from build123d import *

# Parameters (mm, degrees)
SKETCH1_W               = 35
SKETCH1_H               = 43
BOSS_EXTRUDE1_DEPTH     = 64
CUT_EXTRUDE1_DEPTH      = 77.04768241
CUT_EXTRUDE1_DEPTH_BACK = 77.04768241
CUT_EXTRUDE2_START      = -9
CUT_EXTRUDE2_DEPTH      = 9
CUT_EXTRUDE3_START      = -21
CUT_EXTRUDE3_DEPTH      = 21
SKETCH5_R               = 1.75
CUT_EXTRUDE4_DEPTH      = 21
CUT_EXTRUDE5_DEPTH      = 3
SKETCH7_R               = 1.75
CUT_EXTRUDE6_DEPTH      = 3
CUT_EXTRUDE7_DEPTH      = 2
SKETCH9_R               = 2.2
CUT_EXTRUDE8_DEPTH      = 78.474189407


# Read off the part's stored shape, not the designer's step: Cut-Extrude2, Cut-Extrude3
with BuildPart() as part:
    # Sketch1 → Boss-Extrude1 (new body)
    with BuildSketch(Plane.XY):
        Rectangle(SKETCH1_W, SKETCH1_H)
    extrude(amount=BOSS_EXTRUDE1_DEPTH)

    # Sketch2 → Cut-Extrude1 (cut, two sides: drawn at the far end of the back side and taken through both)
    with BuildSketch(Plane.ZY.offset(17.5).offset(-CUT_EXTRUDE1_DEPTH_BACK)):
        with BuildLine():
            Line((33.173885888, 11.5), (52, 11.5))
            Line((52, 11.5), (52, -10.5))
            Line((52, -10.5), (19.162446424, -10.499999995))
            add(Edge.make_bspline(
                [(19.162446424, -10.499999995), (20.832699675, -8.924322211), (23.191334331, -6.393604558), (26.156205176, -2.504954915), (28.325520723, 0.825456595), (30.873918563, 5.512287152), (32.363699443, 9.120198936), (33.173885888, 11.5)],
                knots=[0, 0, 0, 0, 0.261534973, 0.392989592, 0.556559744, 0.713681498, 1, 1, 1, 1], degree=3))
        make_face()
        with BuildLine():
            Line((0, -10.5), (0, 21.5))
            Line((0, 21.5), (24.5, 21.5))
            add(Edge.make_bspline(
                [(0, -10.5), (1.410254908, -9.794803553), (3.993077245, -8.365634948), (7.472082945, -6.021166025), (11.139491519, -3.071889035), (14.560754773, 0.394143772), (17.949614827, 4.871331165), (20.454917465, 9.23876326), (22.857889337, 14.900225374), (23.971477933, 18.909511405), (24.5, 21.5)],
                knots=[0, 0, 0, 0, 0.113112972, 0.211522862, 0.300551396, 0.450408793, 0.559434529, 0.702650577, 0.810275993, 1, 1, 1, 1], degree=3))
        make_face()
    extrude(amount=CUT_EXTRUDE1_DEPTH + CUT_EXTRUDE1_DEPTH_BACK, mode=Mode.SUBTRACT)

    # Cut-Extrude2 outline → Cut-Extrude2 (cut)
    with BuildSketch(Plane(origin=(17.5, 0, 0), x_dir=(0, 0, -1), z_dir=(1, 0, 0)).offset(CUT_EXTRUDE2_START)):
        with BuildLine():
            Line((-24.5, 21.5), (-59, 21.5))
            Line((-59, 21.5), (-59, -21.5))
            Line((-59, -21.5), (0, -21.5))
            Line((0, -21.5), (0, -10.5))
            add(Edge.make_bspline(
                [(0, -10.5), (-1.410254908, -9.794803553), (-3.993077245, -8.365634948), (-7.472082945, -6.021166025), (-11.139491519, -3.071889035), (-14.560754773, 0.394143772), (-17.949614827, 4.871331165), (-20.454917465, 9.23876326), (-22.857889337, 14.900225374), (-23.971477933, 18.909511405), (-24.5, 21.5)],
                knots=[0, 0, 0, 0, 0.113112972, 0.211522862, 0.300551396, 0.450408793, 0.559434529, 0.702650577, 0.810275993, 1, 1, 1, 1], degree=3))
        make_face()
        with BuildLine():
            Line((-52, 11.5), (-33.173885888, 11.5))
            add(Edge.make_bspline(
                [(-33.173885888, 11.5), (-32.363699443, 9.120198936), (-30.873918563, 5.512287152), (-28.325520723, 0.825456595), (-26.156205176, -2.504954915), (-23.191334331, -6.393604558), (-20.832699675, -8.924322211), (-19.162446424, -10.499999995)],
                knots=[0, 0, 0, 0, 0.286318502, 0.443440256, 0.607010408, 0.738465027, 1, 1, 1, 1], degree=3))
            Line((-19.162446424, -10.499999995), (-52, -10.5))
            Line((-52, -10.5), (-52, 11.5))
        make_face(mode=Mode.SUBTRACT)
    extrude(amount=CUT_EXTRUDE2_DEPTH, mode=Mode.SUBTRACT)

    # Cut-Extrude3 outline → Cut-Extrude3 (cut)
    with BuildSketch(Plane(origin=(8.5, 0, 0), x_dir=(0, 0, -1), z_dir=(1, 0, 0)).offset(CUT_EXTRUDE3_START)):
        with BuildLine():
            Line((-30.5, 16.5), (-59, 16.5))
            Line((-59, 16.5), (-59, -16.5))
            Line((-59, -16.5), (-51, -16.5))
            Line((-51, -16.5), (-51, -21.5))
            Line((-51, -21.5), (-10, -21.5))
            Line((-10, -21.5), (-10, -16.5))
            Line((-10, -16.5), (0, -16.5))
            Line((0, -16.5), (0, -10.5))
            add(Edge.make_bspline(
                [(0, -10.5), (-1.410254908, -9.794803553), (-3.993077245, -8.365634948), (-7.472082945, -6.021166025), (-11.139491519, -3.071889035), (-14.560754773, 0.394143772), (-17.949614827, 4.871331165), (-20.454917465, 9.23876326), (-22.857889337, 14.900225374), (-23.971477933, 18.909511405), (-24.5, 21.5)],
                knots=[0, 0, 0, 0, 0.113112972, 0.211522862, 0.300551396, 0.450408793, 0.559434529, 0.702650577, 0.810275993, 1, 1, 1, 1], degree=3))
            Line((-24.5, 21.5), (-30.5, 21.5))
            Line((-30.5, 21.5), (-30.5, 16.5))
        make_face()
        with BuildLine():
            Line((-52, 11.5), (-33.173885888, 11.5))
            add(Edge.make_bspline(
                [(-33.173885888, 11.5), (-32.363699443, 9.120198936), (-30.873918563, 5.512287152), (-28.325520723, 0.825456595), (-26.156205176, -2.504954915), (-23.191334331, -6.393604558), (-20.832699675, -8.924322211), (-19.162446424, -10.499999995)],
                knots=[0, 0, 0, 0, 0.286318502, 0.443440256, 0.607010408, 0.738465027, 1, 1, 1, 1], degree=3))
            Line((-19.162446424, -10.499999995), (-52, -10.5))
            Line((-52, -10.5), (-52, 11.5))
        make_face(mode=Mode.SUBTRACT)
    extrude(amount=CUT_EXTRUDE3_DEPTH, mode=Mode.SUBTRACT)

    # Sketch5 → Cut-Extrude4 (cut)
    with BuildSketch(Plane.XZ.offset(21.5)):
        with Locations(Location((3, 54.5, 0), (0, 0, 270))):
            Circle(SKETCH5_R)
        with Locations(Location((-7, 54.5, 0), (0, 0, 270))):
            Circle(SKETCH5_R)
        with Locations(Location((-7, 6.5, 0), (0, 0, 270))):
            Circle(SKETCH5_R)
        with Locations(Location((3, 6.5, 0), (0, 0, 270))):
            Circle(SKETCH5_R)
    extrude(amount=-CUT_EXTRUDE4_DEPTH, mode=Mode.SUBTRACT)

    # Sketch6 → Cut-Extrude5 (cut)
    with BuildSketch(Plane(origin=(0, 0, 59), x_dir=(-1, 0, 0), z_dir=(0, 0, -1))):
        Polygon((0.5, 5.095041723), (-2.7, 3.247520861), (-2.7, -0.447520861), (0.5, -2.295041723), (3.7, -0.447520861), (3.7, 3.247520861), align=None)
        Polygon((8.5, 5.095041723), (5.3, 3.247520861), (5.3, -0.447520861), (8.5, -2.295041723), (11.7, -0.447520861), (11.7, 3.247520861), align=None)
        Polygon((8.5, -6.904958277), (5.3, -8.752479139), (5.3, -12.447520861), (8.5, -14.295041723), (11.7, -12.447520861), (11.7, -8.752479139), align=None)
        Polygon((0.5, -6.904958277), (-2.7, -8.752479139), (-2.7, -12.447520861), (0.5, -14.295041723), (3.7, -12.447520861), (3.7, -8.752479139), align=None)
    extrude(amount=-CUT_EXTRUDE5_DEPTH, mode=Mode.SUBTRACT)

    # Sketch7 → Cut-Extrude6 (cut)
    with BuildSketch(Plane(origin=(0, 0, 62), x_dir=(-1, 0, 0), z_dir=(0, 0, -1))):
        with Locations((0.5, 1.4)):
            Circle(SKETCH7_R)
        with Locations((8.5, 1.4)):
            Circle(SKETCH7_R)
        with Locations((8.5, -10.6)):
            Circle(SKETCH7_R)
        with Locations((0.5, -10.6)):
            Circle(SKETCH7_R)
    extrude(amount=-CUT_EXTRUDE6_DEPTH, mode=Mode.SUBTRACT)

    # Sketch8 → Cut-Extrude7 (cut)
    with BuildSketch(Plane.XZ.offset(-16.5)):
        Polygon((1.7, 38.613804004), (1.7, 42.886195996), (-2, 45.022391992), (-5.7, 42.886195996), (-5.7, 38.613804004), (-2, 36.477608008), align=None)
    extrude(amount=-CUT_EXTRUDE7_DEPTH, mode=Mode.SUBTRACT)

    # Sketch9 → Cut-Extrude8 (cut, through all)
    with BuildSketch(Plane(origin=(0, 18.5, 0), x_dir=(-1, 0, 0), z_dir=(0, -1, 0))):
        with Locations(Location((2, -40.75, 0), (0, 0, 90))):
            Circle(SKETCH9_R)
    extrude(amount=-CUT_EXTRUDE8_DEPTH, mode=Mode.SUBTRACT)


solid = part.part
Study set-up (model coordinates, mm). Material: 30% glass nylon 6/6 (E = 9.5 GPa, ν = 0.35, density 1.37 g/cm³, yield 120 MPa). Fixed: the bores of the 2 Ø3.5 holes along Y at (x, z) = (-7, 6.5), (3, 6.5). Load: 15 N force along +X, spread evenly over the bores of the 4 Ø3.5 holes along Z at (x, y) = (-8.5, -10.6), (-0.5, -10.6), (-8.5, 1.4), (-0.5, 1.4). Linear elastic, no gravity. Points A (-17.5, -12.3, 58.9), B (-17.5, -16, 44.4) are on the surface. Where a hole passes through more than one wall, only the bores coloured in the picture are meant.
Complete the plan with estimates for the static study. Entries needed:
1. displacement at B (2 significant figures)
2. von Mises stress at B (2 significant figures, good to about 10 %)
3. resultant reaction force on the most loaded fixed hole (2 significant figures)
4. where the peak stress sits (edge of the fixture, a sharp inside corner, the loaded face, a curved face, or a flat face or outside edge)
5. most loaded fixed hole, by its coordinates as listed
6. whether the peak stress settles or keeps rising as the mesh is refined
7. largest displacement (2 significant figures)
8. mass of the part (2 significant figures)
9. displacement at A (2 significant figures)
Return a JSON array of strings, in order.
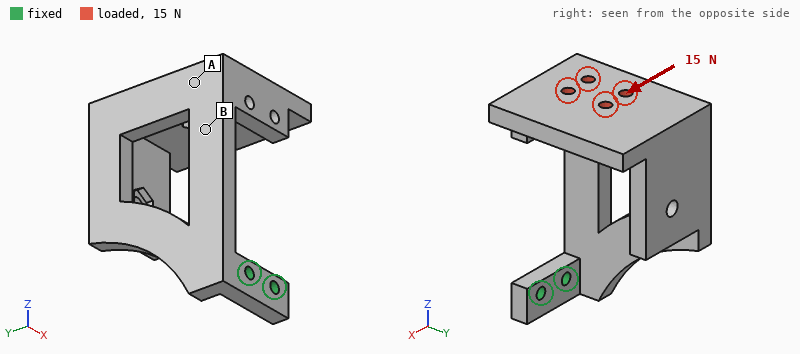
["0.38 mm", "2.7 MPa", "65 N", "a sharp inside corner", "(-7, 6.5)", "keeps rising", "0.96 mm", "26 g", "0.61 mm"]
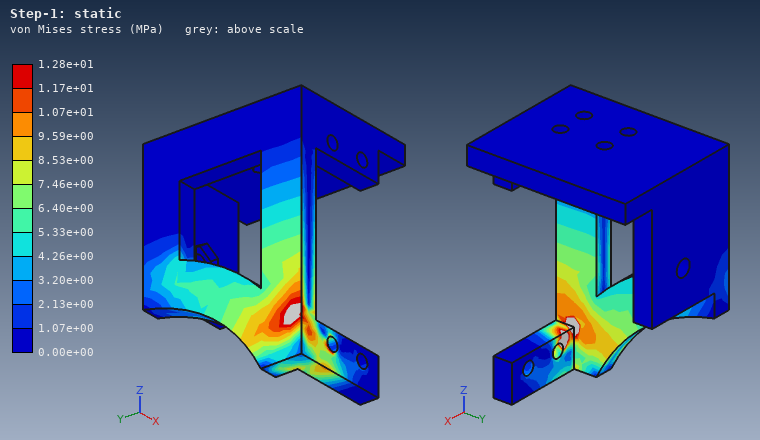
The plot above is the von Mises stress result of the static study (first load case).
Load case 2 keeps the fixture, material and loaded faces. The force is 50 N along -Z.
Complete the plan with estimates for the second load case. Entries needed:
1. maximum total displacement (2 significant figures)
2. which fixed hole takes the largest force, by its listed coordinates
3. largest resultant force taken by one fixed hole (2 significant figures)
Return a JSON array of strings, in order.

["0.85 mm", "(-7, 6.5)", "43 N"]
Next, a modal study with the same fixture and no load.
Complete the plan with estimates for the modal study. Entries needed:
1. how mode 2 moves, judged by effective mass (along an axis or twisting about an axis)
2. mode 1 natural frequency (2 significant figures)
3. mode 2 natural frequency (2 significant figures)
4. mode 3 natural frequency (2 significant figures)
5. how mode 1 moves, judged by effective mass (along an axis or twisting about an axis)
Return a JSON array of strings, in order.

["along Y", "170 Hz", "230 Hz", "450 Hz", "along X"]
